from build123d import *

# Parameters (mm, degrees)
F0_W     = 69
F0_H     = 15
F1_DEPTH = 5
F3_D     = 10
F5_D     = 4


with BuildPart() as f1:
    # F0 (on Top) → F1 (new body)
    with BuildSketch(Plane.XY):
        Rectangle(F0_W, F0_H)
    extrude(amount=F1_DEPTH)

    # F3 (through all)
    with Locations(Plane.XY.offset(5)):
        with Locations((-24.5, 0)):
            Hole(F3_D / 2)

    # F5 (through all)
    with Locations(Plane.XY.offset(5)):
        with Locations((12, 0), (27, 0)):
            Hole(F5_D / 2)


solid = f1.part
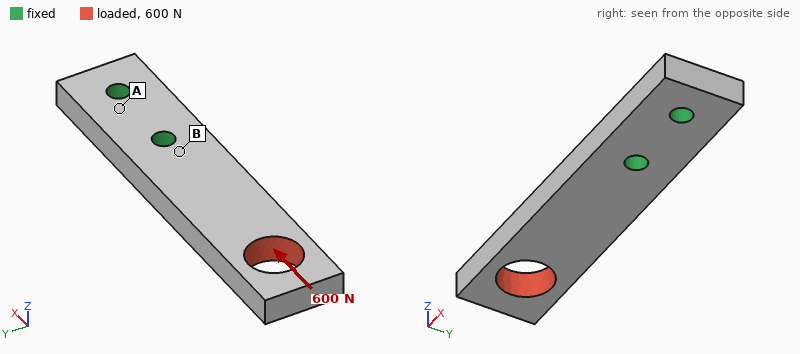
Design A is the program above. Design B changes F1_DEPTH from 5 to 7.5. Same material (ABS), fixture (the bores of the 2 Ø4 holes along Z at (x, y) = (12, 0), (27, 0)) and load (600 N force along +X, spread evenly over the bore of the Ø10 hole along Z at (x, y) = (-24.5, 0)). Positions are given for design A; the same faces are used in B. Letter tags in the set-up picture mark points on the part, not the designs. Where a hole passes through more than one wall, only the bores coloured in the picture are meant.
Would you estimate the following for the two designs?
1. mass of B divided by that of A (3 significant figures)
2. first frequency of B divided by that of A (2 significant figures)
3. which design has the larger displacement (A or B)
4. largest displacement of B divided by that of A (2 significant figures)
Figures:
1.50
1.5
A
0.67
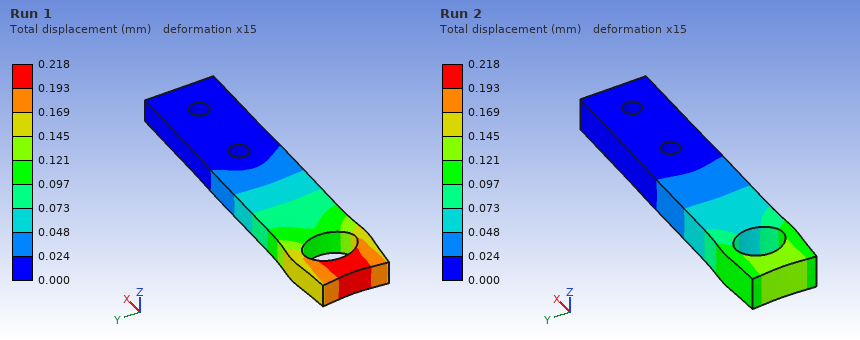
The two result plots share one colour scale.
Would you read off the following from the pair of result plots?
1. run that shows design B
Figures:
Run 2
